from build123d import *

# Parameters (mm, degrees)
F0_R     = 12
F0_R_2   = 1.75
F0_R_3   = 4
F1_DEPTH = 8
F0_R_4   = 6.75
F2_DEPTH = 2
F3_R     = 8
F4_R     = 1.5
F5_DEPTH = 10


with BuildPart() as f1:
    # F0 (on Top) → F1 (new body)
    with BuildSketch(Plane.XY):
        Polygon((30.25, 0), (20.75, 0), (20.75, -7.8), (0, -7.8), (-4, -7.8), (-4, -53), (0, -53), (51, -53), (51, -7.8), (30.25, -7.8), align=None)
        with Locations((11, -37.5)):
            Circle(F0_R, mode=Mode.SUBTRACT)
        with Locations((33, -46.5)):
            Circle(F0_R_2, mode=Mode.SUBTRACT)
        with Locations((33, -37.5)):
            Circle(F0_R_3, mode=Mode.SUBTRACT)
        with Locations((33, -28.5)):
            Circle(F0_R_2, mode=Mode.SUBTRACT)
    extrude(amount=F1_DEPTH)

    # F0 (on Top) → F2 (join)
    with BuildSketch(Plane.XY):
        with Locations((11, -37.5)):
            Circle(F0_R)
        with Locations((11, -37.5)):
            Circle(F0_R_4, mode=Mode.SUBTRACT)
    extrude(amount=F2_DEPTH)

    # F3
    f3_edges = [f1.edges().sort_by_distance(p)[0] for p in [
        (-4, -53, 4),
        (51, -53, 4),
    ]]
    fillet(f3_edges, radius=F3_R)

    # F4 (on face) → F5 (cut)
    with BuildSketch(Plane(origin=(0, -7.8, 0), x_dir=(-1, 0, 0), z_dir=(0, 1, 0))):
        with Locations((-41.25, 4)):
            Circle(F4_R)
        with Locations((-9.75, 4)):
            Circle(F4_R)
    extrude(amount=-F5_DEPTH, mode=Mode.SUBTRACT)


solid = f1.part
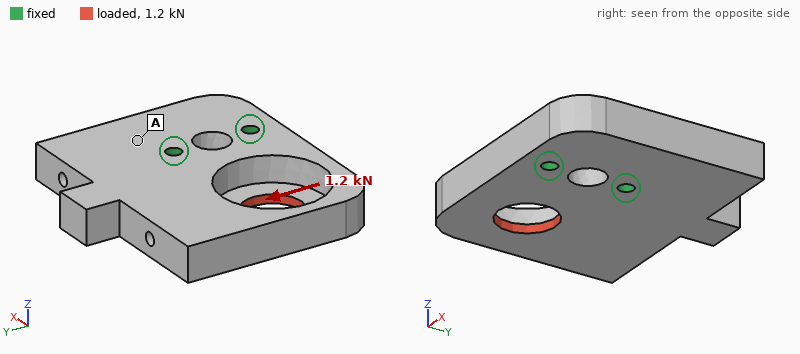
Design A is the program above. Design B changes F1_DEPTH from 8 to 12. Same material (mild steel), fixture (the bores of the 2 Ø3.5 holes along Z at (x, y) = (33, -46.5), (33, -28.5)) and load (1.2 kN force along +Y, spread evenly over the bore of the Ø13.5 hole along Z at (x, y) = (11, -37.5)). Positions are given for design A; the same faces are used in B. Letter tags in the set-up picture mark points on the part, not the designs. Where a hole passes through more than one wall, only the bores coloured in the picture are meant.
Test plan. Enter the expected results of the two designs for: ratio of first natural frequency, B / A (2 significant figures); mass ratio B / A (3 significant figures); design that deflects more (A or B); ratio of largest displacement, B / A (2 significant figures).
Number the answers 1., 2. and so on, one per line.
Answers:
1. 1.4
2. 1.49
3. A
4. 0.73
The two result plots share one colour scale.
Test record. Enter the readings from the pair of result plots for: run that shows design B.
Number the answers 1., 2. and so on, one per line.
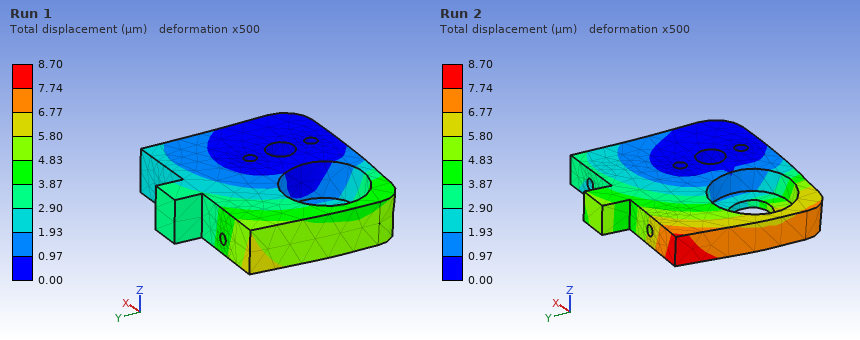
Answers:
1. Run 1
